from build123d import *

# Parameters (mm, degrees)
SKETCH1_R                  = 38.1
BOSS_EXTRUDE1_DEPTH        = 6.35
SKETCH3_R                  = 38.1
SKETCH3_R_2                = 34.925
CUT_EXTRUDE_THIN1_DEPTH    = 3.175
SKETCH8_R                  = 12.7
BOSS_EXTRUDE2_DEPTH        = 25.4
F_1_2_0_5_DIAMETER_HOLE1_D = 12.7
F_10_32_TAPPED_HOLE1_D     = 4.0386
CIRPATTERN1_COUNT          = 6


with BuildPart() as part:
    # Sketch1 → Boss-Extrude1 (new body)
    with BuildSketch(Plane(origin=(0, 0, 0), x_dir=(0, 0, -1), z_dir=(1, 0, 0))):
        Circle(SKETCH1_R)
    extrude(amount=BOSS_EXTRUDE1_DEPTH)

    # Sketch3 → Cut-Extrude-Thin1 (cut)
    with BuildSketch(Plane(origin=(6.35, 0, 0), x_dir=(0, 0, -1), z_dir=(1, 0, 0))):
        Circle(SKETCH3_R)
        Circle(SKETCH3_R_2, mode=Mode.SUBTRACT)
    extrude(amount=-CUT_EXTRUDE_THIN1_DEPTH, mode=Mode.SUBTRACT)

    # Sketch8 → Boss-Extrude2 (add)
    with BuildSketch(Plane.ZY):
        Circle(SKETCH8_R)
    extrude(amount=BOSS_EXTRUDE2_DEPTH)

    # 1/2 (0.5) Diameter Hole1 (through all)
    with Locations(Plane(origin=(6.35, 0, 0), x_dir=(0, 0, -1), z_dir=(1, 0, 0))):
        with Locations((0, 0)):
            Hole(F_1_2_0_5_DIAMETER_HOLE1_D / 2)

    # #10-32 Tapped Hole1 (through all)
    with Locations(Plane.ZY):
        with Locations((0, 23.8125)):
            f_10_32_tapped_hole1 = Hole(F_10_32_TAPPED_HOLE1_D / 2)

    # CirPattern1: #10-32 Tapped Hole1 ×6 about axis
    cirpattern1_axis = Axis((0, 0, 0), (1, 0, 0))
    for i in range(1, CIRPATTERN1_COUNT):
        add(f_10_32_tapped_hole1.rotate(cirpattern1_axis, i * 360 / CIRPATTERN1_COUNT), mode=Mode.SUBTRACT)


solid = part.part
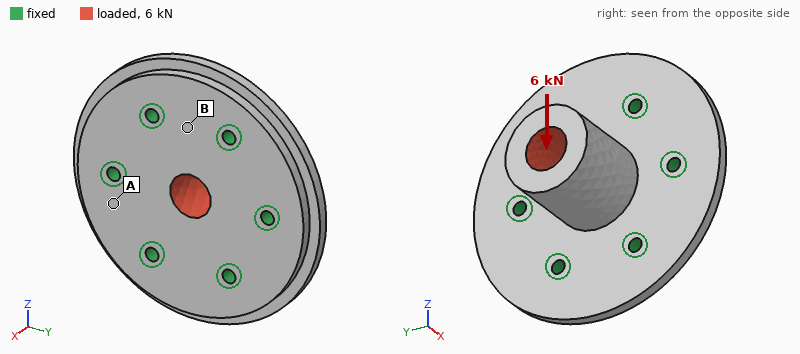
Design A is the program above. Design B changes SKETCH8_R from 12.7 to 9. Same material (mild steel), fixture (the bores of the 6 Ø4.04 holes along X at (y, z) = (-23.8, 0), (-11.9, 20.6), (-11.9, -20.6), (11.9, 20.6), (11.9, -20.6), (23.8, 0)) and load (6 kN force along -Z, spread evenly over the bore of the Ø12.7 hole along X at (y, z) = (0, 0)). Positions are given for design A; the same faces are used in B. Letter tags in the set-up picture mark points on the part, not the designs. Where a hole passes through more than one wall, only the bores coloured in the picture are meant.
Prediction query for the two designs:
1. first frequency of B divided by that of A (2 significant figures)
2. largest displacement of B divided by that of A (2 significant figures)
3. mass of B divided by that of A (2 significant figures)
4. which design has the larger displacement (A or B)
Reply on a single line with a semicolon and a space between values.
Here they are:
0.97; 3.1; 0.82; B
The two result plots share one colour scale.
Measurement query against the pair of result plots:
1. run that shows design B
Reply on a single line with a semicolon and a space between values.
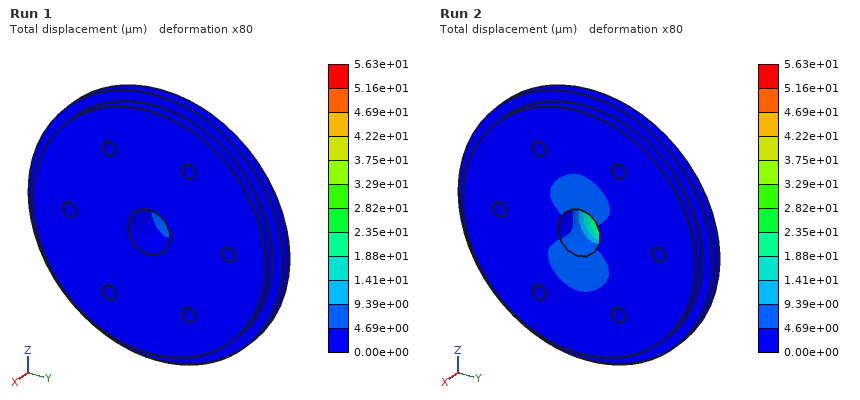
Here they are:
Run 2
